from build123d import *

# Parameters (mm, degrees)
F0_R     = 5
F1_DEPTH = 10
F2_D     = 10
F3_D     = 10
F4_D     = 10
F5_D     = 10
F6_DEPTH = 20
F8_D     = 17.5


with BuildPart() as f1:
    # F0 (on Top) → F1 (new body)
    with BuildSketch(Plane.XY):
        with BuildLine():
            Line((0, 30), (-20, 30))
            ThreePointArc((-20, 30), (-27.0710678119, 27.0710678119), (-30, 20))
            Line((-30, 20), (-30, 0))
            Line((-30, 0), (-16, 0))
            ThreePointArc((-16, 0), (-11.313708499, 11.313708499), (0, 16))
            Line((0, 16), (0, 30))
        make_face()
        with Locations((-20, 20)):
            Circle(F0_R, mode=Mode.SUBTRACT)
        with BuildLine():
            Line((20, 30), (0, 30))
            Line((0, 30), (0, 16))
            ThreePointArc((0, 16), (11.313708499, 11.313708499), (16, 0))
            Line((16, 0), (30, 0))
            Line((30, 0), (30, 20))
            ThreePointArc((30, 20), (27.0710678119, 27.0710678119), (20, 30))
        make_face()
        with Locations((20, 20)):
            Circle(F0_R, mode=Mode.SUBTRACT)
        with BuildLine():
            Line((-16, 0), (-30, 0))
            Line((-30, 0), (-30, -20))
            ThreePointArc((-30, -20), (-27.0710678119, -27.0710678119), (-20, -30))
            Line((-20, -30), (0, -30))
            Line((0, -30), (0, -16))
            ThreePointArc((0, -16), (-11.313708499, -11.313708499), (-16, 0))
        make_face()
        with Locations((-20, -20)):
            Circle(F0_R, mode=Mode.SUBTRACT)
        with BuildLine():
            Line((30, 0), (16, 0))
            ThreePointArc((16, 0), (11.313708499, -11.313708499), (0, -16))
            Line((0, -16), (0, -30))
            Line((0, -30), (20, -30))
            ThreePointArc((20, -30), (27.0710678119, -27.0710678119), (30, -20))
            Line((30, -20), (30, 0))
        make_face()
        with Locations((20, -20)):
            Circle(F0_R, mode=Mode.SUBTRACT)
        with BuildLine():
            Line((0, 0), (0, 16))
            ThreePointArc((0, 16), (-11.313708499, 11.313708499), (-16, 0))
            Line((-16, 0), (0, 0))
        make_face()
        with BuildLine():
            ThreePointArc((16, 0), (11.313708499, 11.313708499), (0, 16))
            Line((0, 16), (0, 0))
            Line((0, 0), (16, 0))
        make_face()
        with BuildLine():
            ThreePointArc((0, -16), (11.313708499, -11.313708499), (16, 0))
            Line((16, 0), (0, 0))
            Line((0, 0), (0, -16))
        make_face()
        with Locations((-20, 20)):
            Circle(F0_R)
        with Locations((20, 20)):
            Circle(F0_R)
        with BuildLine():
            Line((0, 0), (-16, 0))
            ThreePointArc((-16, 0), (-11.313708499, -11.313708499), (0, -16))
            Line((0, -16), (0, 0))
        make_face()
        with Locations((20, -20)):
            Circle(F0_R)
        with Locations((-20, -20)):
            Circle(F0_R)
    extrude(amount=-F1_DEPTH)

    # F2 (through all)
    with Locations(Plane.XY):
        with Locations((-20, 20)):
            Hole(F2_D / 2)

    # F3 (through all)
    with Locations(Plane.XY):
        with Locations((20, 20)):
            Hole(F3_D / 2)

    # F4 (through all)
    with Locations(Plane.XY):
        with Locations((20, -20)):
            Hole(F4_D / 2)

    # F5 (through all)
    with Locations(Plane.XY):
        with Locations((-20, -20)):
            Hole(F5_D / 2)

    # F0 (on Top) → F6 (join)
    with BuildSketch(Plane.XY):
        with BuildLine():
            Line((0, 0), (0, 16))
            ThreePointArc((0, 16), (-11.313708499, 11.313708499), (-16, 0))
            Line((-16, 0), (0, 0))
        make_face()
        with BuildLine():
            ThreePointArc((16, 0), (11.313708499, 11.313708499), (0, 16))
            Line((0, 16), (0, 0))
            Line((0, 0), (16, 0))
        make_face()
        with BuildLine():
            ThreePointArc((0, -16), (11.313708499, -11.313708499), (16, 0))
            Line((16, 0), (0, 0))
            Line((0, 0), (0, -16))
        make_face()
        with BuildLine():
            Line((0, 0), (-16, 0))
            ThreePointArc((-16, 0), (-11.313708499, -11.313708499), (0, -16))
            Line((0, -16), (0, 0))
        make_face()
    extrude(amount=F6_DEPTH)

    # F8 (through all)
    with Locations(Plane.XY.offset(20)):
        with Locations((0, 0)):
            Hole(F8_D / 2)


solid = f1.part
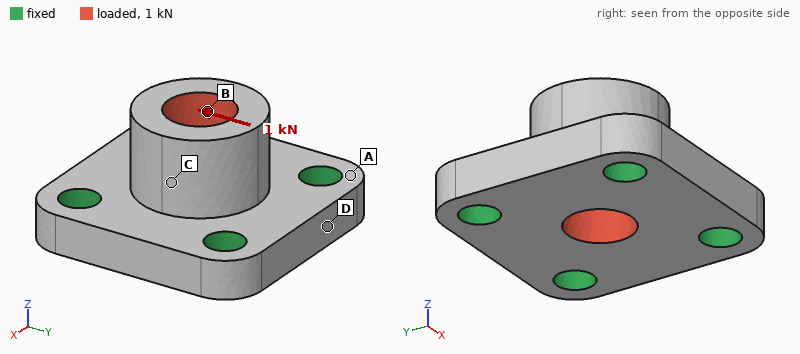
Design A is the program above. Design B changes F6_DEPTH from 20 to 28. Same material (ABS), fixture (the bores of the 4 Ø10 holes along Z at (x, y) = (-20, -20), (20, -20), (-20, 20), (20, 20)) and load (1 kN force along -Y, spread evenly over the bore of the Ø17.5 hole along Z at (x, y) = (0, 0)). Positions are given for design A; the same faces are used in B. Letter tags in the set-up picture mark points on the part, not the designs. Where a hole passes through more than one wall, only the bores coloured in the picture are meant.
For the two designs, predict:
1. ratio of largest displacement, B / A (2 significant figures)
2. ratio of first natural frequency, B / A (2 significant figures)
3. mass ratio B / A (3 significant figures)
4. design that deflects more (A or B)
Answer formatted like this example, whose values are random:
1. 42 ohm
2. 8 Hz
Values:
1. 1.7
2. 0.69
3. 1.11
4. B
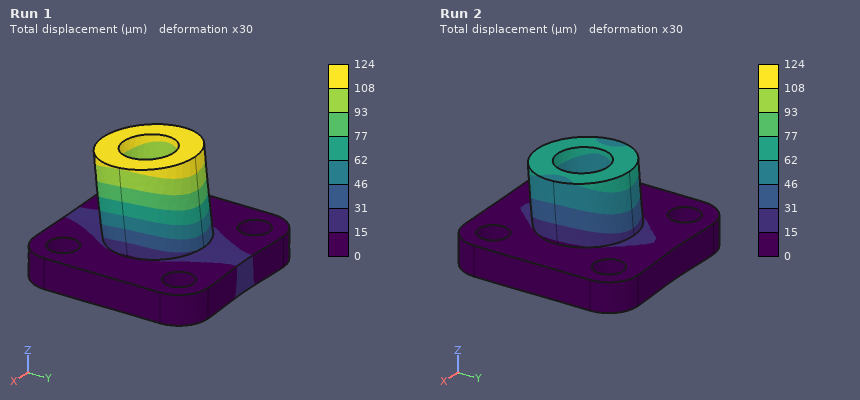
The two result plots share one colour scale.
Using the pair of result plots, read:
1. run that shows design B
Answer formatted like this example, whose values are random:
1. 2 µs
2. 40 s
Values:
1. Run 1
